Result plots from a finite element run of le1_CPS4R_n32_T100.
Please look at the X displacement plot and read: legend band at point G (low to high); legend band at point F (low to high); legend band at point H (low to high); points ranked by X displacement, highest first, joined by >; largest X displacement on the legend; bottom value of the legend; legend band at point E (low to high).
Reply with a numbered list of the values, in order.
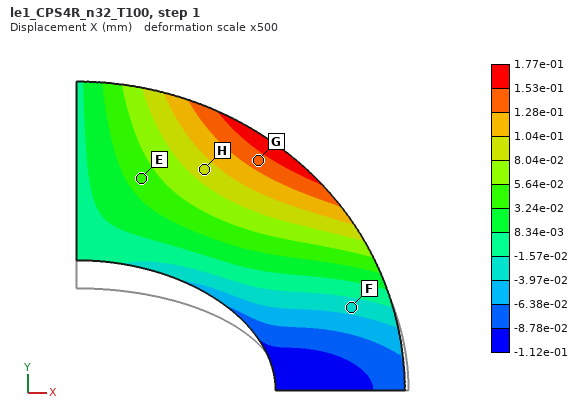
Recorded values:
1. 1.28e-01 to 1.53e-01 mm
2. -3.97e-02 to -1.57e-02 mm
3. 8.04e-02 to 1.04e-01 mm
4. G > H > E > F
5. 1.77e-01 mm
6. -1.12e-01 mm
7. 3.24e-02 to 5.64e-02 mm
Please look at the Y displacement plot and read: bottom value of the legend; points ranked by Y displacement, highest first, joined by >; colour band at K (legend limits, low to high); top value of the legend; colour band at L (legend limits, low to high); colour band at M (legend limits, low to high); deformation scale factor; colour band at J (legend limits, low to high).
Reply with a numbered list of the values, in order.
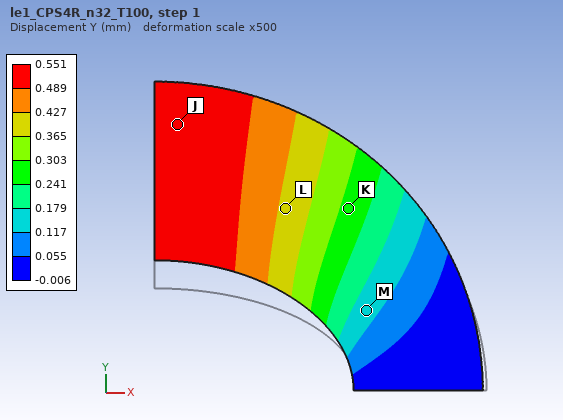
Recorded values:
1. -0.006 mm
2. J > L > K > M
3. 0.241 to 0.303 mm
4. 0.551 mm
5. 0.365 to 0.427 mm
6. 0.117 to 0.179 mm
7. 500
8. 0.489 to 0.551 mm
